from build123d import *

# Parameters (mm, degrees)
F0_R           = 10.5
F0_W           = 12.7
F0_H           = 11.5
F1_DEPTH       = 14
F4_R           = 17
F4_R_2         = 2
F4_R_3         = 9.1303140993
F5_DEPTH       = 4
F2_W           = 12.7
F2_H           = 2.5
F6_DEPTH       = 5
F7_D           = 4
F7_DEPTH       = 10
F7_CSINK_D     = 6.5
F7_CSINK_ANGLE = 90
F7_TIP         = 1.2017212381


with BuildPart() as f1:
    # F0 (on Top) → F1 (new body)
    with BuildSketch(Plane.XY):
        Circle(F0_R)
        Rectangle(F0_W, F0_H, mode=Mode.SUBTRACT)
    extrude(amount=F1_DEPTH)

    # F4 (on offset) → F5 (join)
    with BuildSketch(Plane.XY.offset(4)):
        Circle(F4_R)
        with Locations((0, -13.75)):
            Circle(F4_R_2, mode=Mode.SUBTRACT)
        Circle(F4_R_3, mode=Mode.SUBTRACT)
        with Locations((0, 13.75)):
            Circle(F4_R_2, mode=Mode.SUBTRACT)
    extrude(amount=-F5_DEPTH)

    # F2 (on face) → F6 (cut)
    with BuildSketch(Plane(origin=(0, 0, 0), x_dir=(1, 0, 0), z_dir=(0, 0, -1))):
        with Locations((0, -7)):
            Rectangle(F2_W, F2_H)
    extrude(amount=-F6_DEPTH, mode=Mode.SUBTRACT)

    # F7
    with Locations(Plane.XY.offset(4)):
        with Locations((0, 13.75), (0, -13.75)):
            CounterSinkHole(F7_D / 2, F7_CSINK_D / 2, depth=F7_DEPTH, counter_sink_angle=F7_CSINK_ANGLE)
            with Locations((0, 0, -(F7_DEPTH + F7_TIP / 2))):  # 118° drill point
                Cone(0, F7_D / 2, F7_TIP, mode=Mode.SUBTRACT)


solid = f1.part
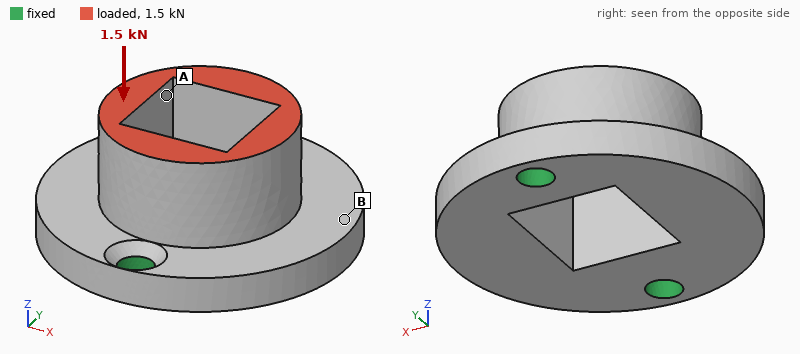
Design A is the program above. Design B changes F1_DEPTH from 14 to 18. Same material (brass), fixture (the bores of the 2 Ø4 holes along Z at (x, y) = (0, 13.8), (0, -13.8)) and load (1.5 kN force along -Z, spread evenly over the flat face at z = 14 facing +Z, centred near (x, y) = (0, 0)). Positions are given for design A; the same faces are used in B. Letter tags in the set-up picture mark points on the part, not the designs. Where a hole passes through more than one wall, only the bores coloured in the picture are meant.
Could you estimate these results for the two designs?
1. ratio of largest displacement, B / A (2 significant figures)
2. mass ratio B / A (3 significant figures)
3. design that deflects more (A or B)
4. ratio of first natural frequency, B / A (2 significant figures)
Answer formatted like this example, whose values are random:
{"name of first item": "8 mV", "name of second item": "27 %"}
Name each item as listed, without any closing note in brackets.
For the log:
{"ratio of largest displacement, B / A": "0.85", "mass ratio B / A": "1.17", "design that deflects more": "A", "ratio of first natural frequency, B / A": "0.83"}
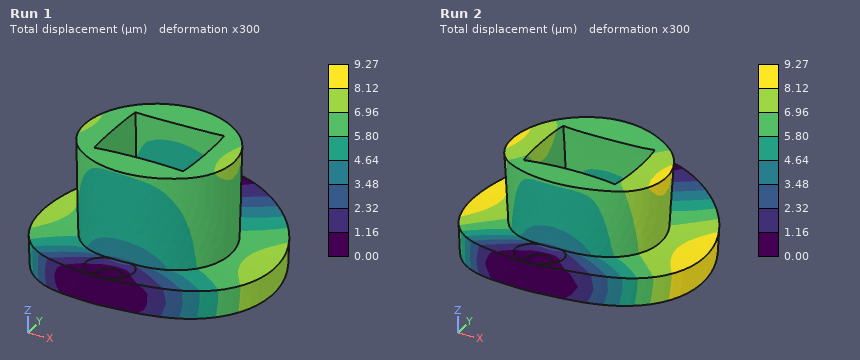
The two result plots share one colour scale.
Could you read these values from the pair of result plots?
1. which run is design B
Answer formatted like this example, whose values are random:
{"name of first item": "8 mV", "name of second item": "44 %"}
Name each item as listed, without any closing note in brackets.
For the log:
{"which run is design B": "Run 1"}
